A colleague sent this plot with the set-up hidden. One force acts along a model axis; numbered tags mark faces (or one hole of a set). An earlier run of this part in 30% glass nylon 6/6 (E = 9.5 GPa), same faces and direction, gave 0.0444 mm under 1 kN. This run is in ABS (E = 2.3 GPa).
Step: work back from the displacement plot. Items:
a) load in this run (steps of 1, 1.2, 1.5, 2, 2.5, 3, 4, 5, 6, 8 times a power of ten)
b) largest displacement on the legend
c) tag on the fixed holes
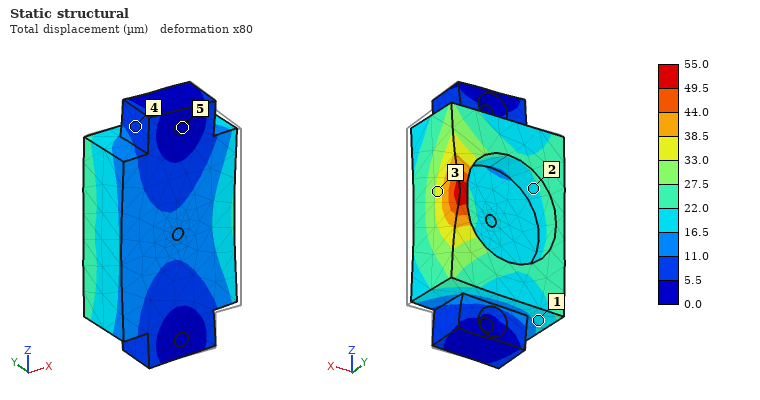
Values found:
300 N
55.0 µm
5
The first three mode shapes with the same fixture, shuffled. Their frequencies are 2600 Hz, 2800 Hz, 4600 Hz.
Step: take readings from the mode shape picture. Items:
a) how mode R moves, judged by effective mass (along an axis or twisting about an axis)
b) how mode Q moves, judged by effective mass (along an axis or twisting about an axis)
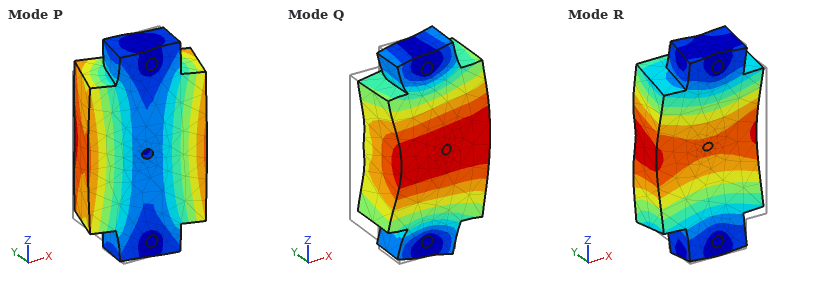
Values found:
along Y
along X
